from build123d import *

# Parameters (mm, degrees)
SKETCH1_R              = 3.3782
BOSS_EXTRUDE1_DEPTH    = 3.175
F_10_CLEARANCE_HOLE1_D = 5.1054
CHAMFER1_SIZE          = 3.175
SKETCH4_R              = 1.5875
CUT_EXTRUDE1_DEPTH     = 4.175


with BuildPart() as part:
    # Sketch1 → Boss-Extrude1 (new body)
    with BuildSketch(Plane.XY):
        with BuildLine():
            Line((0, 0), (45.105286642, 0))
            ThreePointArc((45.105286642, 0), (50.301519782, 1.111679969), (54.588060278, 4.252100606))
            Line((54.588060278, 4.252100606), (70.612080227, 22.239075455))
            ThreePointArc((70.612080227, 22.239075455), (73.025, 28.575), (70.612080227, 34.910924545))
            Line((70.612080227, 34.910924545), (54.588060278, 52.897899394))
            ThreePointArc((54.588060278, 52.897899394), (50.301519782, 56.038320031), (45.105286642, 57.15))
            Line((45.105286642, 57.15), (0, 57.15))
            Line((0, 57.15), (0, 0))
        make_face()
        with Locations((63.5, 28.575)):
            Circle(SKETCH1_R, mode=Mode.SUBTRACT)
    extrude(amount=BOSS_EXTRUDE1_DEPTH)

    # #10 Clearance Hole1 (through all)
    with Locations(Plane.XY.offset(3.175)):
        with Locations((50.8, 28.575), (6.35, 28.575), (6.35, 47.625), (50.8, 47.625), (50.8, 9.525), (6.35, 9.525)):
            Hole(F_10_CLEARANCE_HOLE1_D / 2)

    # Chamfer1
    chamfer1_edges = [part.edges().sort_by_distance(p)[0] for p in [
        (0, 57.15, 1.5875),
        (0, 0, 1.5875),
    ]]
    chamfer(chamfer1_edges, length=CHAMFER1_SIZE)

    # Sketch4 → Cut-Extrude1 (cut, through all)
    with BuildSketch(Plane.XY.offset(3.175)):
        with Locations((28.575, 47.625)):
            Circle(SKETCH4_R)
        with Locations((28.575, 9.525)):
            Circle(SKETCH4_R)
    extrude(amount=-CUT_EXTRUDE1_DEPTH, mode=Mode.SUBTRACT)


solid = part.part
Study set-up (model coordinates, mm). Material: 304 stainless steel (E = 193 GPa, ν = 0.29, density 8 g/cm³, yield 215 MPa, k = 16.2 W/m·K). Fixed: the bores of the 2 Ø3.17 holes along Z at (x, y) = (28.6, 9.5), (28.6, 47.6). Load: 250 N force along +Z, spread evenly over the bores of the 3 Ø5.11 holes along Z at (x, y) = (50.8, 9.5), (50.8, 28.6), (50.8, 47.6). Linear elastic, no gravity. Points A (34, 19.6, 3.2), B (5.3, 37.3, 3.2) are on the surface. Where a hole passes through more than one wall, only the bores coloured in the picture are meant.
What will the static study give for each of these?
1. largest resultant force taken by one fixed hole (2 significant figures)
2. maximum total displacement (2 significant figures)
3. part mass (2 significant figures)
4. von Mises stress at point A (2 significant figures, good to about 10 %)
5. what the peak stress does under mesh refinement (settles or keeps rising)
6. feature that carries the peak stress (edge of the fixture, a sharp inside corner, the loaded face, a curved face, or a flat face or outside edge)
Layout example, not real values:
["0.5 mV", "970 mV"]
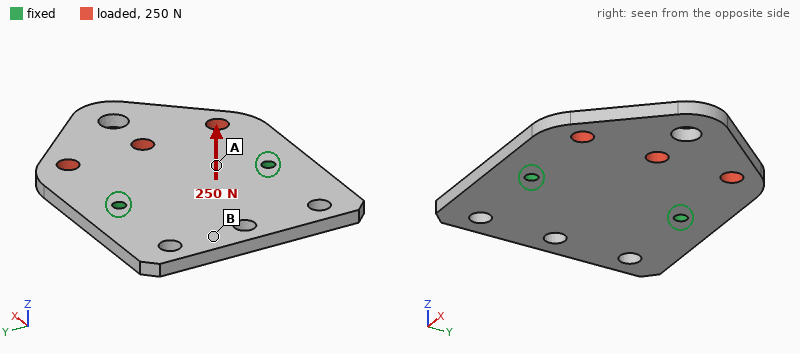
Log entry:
["130 N", "100 µm", "87 g", "33 MPa", "keeps rising", "edge of the fixture"]
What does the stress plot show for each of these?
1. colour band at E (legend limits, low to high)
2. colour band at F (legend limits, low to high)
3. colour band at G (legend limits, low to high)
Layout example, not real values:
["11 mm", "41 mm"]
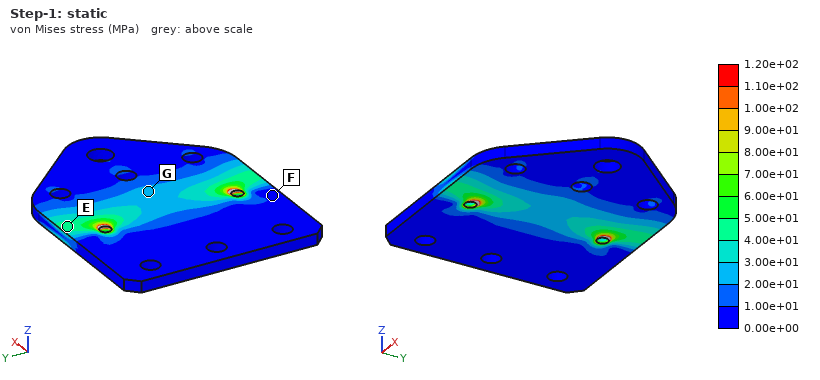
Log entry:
["4.00e+01 to 5.00e+01 MPa", "0.00e+00 to 1.00e+01 MPa", "2.00e+01 to 3.00e+01 MPa"]
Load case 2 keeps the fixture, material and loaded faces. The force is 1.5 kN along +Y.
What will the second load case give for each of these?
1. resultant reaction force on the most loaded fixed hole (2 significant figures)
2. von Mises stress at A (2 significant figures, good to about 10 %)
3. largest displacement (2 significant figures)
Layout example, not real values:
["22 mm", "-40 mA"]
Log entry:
["1.1 kN", "18 MPa", "6.0 µm"]
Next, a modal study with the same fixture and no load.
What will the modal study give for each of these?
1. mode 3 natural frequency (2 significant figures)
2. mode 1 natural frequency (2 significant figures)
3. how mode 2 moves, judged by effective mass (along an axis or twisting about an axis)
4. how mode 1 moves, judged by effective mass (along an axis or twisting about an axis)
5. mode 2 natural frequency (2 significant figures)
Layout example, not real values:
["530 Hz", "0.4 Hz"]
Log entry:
["4400 Hz", "1700 Hz", "along Z", "along Z", "2900 Hz"]
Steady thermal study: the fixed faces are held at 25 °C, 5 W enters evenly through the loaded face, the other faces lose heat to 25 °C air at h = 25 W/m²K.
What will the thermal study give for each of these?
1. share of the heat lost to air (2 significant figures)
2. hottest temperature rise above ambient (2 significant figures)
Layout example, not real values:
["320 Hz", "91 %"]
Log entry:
["49 %", "34 K"]
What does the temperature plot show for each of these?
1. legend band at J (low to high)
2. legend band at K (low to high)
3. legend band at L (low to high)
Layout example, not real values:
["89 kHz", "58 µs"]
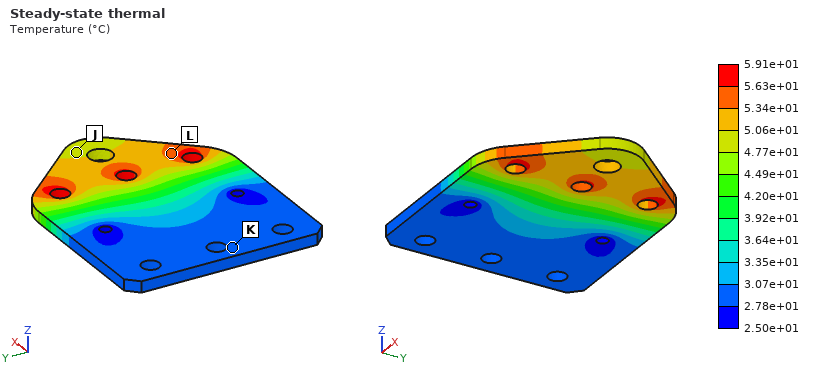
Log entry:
["4.77e+01 to 5.06e+01 °C", "2.78e+01 to 3.07e+01 °C", "5.34e+01 to 5.63e+01 °C"]
